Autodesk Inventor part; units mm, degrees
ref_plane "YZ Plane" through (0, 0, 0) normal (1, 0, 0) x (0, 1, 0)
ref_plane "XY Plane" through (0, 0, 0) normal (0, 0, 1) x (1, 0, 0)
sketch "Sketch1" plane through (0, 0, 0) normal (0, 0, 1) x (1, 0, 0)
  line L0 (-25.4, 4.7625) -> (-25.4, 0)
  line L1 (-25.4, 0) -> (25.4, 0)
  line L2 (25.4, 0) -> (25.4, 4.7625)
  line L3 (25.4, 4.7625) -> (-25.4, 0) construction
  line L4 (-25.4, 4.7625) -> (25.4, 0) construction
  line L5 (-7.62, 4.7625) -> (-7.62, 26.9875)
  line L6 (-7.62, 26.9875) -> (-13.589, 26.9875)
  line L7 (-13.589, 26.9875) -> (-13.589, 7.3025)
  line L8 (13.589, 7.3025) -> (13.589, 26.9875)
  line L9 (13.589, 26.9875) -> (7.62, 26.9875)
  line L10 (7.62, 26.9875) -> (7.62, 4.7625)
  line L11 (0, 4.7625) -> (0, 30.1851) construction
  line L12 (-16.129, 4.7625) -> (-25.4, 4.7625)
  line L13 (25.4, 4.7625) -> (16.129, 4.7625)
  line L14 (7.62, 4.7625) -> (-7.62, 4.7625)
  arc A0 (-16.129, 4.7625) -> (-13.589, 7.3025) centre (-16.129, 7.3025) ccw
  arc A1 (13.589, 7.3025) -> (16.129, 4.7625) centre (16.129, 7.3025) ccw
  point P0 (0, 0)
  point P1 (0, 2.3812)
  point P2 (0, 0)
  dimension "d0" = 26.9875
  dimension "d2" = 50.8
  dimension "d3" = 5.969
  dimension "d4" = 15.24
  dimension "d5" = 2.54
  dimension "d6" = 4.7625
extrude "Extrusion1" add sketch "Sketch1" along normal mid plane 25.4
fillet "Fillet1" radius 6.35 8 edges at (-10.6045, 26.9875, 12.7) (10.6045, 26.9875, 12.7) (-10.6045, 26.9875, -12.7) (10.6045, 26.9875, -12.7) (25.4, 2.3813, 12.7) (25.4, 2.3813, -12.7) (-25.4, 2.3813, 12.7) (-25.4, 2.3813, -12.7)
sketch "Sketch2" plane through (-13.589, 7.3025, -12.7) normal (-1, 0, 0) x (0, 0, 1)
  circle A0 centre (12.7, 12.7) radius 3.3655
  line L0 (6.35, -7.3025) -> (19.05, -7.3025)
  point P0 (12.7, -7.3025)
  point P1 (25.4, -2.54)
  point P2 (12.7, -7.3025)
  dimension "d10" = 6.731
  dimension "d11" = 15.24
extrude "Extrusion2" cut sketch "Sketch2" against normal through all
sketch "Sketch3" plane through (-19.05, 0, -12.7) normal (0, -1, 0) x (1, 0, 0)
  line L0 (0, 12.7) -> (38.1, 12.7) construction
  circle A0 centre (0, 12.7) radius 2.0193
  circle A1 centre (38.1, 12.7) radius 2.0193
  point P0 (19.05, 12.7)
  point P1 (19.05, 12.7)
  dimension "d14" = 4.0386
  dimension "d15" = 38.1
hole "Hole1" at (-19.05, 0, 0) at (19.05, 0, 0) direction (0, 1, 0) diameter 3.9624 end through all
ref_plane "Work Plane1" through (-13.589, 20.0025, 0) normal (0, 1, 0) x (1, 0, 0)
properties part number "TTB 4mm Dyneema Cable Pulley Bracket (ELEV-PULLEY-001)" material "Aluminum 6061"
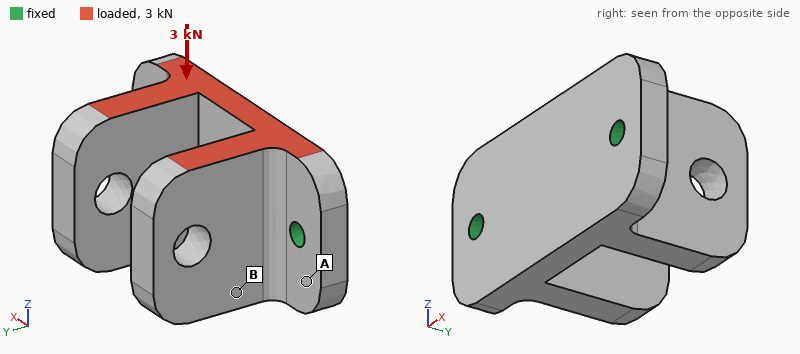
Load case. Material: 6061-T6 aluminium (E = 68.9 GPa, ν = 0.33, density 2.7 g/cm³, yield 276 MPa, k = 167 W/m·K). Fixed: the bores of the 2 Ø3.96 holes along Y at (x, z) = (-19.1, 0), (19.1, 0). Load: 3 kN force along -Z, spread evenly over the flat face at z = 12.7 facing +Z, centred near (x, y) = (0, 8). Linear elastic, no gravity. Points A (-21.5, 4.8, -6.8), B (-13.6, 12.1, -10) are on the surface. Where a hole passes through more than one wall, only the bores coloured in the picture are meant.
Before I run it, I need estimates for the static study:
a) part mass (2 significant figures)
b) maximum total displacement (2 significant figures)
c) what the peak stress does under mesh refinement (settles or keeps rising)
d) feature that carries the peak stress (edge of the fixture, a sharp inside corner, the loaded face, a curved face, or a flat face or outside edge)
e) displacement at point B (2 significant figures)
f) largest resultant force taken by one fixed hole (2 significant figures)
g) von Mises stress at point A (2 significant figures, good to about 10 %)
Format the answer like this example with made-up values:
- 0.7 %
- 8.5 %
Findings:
- 33 g
- 70 µm
- keeps rising
- edge of the fixture
- 38 µm
- 1.5 kN
- 29 MPa
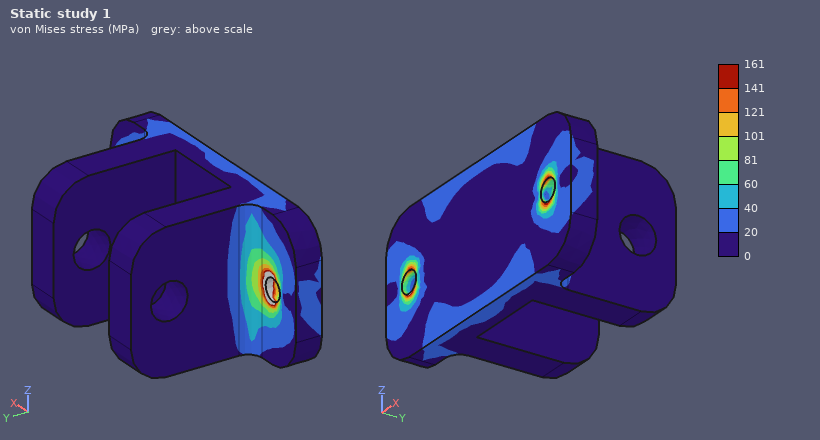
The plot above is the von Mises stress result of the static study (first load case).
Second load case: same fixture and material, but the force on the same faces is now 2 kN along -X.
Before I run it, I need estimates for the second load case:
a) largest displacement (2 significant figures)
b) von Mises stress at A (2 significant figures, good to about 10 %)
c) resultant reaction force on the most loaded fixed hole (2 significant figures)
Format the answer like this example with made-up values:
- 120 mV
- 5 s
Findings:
- 35 µm
- 4.8 MPa
- 1.2 kN
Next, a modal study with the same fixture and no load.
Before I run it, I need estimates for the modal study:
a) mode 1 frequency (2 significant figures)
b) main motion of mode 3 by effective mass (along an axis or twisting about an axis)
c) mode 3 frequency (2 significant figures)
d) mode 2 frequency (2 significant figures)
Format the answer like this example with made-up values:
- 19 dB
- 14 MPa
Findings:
- 5600 Hz
- along X
- 8300 Hz
- 5600 Hz
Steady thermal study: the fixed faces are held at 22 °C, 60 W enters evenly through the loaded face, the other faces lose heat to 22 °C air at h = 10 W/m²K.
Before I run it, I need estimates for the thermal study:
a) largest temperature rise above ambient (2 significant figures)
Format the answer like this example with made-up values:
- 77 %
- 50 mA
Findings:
- 26 K
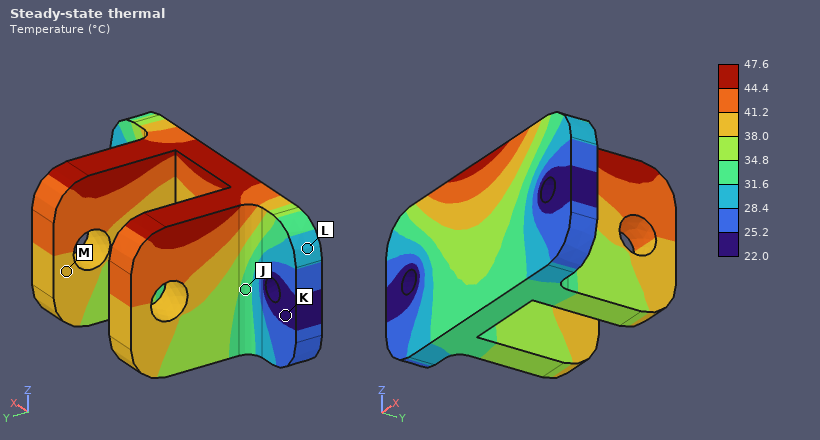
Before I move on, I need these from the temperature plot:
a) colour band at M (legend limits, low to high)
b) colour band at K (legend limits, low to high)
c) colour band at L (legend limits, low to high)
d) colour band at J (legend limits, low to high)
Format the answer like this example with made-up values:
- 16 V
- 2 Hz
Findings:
- 38.0 to 41.2 °C
- 22.0 to 25.2 °C
- 28.4 to 31.6 °C
- 31.6 to 34.8 °C
